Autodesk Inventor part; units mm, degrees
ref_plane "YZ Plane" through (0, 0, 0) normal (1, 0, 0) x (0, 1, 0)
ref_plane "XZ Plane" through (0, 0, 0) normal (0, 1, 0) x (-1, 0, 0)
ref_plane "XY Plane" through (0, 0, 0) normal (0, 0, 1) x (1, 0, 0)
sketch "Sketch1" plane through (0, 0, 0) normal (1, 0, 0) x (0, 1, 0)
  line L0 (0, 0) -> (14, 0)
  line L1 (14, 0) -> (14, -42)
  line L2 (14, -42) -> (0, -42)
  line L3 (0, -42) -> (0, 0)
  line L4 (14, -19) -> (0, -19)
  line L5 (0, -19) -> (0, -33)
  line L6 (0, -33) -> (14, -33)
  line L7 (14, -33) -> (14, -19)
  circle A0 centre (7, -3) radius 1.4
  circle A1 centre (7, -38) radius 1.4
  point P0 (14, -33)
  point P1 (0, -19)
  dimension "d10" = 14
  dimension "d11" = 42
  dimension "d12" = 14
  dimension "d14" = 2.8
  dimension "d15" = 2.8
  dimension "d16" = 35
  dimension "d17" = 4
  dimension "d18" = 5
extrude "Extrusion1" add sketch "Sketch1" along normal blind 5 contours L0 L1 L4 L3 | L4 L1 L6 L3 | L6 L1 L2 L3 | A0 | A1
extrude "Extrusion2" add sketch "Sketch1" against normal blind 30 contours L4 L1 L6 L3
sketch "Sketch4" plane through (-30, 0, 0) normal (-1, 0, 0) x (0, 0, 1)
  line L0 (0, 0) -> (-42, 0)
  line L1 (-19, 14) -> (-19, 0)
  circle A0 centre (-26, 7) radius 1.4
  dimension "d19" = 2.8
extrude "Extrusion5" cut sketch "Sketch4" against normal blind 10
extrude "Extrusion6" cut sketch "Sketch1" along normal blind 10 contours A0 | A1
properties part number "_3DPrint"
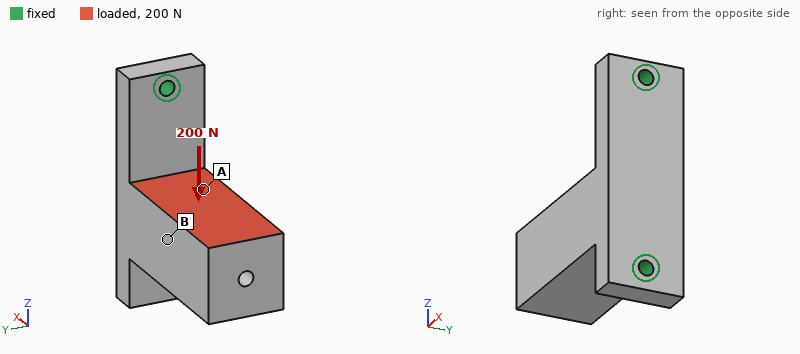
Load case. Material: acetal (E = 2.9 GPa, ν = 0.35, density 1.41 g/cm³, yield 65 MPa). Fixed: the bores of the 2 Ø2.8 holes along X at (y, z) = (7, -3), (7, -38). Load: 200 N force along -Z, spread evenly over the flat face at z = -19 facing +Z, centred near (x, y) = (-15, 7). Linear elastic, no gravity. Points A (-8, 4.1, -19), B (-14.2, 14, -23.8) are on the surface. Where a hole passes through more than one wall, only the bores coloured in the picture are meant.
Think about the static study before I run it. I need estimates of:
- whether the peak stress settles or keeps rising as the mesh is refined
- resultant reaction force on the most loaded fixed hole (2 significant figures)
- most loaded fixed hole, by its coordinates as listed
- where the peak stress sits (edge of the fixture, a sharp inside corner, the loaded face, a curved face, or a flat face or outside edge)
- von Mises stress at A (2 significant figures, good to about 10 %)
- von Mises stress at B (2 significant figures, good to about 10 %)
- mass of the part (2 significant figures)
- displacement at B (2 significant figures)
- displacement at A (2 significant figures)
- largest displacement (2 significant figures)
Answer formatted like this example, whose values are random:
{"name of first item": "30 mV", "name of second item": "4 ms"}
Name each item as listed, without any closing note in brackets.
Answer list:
{"whether the peak stress settles or keeps rising as the mesh is refined": "keeps rising", "resultant reaction force on the most loaded fixed hole": "170 N", "most loaded fixed hole, by its coordinates as listed": "(7, -38)", "where the peak stress sits": "edge of the fixture", "von Mises stress at A": "3.7 MPa", "von Mises stress at B": "1.7 MPa", "mass of the part": "12 g", "displacement at B": "0.21 mm", "displacement at A": "0.18 mm", "largest displacement": "0.41 mm"}
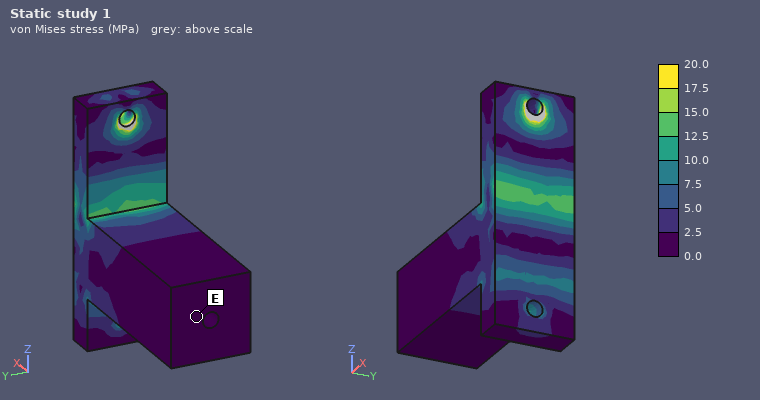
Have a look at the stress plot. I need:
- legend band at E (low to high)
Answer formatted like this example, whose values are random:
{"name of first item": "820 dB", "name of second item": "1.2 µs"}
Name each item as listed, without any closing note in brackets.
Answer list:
{"legend band at E": "0.0 to 2.5 MPa"}
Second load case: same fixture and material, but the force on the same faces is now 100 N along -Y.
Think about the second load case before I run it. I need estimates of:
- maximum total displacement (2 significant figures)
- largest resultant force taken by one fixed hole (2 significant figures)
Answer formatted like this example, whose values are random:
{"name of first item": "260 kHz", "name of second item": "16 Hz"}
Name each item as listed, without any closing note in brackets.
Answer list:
{"maximum total displacement": "0.63 mm", "largest resultant force taken by one fixed hole": "51 N"}
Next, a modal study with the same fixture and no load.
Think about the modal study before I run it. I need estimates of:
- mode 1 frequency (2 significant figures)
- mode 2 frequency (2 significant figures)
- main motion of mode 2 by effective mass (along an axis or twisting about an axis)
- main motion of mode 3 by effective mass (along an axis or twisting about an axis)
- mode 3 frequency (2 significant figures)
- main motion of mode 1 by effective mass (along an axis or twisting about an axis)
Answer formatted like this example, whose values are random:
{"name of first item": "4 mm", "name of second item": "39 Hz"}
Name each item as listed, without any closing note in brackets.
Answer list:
{"mode 1 frequency": "870 Hz", "mode 2 frequency": "1400 Hz", "main motion of mode 2 by effective mass": "along Z", "main motion of mode 3 by effective mass": "along X", "mode 3 frequency": "3500 Hz", "main motion of mode 1 by effective mass": "along Y"}
